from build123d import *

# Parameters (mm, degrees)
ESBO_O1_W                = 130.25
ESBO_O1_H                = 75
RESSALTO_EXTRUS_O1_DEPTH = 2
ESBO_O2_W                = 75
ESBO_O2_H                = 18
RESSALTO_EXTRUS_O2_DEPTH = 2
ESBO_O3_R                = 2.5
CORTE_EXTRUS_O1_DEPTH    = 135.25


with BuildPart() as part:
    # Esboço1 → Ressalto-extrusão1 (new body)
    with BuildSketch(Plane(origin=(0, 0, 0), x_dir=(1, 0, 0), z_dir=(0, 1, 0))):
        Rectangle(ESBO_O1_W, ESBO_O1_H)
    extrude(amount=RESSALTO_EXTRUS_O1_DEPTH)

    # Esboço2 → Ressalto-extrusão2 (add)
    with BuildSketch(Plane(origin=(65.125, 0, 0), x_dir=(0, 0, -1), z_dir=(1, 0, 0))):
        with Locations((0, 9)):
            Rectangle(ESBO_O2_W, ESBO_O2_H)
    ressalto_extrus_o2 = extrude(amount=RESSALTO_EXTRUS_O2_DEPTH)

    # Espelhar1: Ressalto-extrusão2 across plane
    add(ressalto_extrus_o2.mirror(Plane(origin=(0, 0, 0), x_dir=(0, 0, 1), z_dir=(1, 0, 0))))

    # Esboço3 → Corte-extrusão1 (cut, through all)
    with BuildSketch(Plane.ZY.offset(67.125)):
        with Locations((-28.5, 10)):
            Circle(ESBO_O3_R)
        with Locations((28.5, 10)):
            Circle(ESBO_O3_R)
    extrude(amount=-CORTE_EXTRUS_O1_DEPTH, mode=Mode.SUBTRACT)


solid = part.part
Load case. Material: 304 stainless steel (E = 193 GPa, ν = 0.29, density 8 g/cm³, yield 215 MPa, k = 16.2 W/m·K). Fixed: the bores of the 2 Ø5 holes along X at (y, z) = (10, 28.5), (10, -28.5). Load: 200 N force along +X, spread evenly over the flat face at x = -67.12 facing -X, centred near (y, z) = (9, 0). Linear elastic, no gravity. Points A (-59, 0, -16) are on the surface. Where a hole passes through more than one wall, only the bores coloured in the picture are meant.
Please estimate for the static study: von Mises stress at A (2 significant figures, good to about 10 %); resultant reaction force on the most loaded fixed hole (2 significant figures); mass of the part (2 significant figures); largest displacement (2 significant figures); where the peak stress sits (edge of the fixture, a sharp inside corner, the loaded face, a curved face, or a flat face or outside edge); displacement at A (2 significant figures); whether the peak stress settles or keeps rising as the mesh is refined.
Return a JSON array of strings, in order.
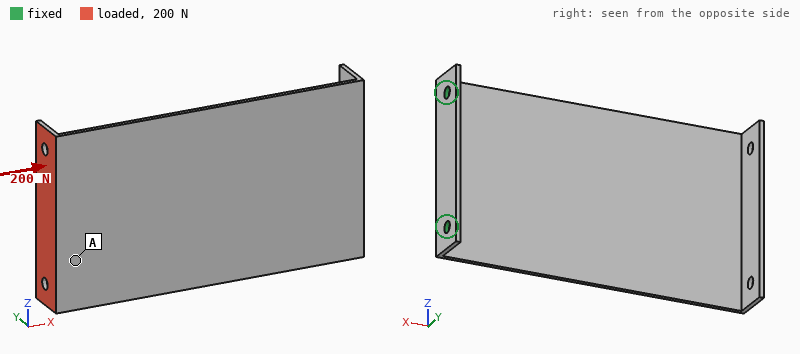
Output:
["27 MPa", "100 N", "200 g", "1.6 mm", "edge of the fixture", "1.3 mm", "keeps rising"]
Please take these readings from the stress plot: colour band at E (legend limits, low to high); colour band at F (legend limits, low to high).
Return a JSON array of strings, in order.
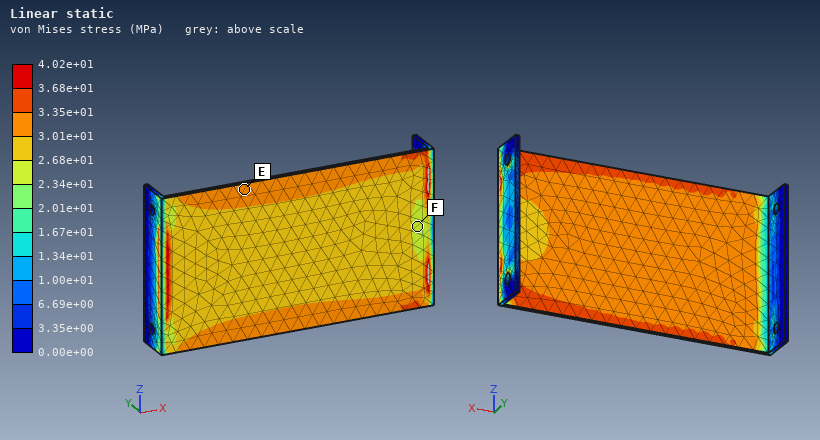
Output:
["3.01e+01 to 3.35e+01 MPa", "2.34e+01 to 2.68e+01 MPa"]
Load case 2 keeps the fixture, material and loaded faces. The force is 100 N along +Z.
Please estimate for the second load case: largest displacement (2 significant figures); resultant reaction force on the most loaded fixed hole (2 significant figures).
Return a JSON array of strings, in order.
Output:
["0.33 mm", "240 N"]
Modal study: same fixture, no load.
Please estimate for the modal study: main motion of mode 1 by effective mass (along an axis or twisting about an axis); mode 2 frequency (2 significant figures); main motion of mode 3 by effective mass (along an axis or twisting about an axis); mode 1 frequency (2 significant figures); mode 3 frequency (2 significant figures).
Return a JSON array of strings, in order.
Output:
["along Y", "290 Hz", "along Y", "66 Hz", "440 Hz"]
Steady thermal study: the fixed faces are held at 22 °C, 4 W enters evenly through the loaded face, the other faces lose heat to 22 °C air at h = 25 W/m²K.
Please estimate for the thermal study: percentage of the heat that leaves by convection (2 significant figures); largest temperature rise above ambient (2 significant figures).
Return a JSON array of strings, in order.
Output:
["100 %", "37 K"]
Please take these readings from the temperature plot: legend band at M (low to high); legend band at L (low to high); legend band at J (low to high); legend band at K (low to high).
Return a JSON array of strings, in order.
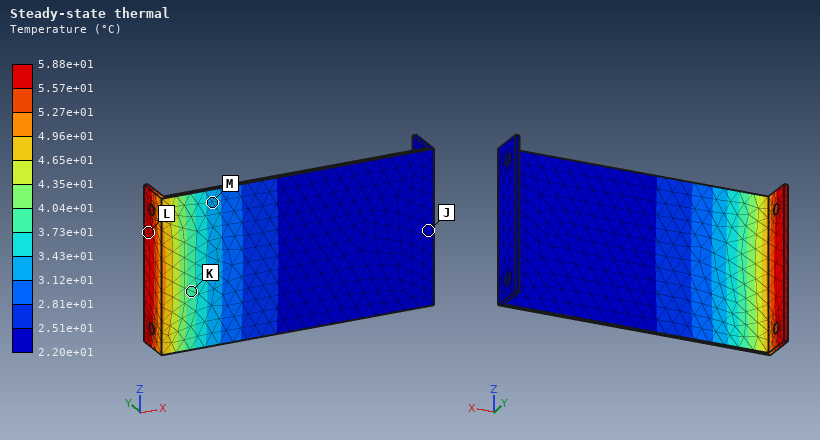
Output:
["3.12e+01 to 3.43e+01 °C", "5.57e+01 to 5.88e+01 °C", "2.20e+01 to 2.51e+01 °C", "3.73e+01 to 4.04e+01 °C"]
